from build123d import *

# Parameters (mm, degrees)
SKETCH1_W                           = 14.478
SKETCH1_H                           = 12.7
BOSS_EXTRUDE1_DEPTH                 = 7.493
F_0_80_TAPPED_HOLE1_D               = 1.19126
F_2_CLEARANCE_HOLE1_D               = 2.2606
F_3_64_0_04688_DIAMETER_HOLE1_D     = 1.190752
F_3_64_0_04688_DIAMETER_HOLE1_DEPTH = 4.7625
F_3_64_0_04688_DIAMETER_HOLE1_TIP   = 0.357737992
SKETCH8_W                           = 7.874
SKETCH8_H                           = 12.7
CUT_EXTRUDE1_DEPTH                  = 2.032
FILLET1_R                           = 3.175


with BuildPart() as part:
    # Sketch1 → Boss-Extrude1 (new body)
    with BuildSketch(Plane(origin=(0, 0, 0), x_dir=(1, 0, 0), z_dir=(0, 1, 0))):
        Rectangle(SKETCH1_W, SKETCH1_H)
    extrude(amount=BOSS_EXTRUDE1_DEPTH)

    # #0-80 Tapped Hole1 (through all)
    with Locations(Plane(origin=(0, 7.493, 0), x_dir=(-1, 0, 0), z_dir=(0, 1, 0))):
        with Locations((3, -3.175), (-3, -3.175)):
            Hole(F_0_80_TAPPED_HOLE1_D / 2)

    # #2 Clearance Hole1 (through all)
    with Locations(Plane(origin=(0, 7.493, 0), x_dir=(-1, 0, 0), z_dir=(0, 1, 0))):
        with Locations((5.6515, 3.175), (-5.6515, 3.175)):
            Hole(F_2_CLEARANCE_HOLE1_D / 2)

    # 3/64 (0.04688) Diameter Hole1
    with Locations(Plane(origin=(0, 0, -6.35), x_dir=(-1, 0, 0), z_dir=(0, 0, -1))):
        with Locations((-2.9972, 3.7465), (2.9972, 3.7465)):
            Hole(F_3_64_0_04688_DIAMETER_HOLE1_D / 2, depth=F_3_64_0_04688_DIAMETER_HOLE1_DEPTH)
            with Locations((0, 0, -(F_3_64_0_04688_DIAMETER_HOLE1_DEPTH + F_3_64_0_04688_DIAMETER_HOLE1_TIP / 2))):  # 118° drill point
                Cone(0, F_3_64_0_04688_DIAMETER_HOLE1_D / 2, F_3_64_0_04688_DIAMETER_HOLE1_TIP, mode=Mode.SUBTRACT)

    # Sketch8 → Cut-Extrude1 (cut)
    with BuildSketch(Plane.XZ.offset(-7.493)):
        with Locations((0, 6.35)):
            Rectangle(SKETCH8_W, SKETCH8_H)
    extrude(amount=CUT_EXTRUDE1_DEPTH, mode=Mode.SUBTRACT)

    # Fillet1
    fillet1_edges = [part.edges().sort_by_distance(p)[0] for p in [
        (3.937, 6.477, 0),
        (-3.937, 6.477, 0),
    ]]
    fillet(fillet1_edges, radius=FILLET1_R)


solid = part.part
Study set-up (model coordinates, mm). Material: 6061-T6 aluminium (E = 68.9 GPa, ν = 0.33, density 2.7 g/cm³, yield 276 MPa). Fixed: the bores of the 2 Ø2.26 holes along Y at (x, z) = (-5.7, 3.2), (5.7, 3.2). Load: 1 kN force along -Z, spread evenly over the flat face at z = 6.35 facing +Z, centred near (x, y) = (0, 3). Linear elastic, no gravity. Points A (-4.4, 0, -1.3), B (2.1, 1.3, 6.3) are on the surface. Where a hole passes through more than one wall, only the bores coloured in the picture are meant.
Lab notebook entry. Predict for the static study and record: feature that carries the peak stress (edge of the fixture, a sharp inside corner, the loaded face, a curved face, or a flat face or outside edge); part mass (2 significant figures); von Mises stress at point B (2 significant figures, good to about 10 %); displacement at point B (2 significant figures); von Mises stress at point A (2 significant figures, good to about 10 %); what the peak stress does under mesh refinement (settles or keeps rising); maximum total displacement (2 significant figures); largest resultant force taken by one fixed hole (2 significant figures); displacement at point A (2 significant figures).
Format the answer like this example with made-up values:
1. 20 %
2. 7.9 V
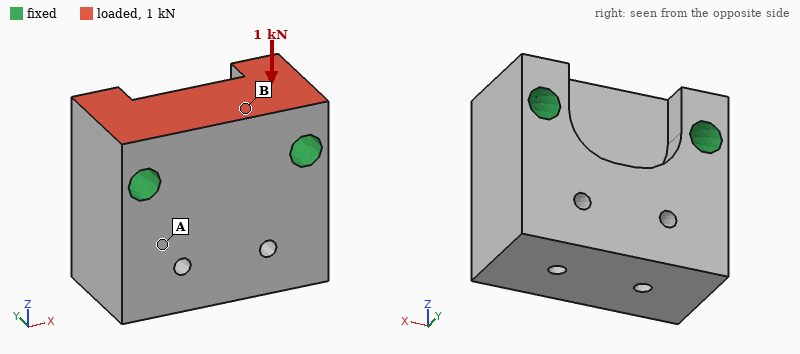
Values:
1. edge of the fixture
2. 3.2 g
3. 10 MPa
4. 1.1 µm
5. 3.7 MPa
6. keeps rising
7. 1.4 µm
8. 500 N
9. 0.38 µm
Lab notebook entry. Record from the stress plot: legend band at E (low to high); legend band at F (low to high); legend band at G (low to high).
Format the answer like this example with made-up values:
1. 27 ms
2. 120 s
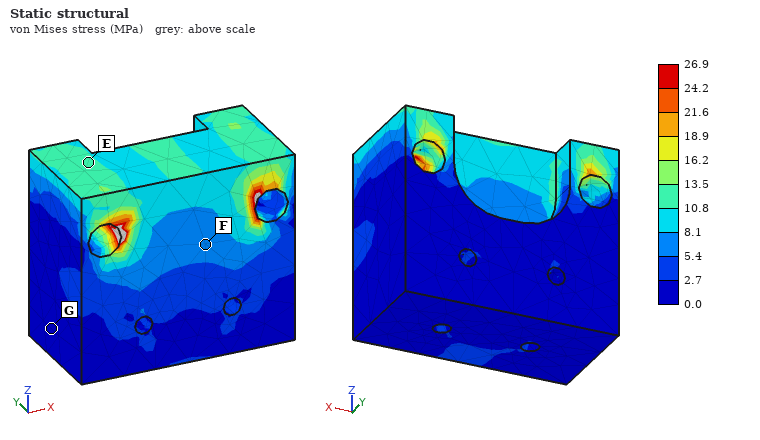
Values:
1. 10.8 to 13.5 MPa
2. 5.4 to 8.1 MPa
3. 0.0 to 2.7 MPa
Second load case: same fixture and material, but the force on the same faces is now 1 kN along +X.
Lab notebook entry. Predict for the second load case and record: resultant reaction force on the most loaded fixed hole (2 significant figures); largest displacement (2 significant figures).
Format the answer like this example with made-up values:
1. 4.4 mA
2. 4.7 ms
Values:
1. 530 N
2. 2.4 µm
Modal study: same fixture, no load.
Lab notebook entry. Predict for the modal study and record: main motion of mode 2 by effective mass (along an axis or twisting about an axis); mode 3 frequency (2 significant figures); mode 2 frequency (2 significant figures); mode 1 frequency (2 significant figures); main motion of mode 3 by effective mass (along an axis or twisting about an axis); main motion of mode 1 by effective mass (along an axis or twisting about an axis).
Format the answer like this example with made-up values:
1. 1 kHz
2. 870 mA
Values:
1. along X
2. 70 kHz
3. 65 kHz
4. 44 kHz
5. along X
6. along Y
